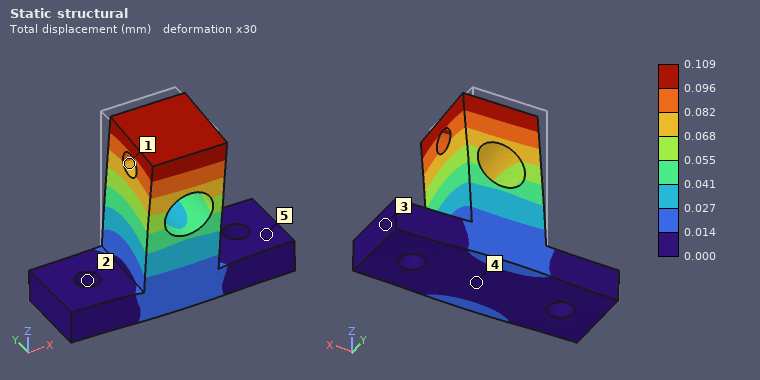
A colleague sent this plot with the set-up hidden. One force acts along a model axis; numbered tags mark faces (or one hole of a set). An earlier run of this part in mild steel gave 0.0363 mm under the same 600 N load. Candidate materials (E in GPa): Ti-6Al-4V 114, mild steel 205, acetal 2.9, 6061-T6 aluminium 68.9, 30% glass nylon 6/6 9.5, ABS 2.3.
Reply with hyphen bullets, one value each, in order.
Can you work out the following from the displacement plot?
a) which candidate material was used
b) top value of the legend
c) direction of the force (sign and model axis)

- 6061-T6 aluminium
- 0.109 mm
- -Y
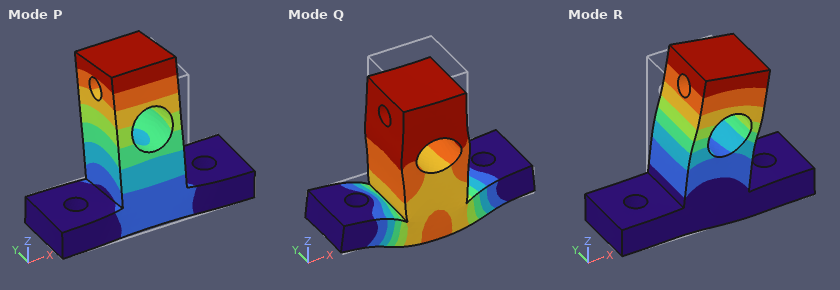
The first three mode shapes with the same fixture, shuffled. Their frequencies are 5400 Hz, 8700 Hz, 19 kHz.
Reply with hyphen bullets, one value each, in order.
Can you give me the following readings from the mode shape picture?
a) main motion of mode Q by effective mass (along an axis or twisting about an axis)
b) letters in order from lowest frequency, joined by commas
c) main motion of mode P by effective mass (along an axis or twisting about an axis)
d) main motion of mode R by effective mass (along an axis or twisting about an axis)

- along Z
- P, R, Q
- along Y
- along X
